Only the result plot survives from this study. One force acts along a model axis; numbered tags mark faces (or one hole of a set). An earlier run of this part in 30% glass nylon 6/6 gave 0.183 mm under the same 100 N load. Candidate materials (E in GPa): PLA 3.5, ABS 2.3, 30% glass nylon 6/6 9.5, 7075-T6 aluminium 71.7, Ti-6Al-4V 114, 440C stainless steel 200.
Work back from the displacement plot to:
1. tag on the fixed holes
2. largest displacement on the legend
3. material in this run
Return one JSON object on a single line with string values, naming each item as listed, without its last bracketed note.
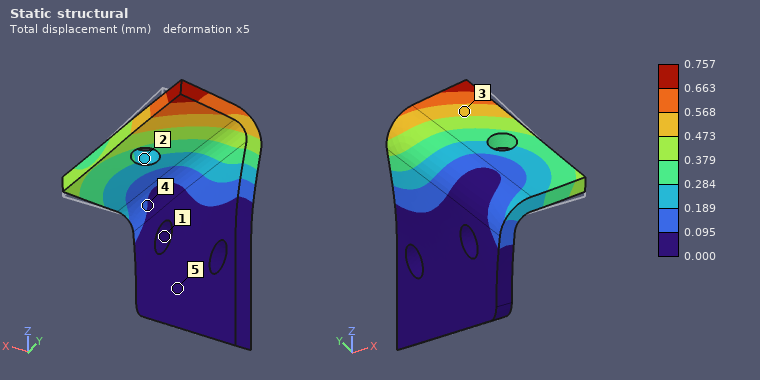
{"tag on the fixed holes": "1", "largest displacement on the legend": "0.757 mm", "material in this run": "ABS"}
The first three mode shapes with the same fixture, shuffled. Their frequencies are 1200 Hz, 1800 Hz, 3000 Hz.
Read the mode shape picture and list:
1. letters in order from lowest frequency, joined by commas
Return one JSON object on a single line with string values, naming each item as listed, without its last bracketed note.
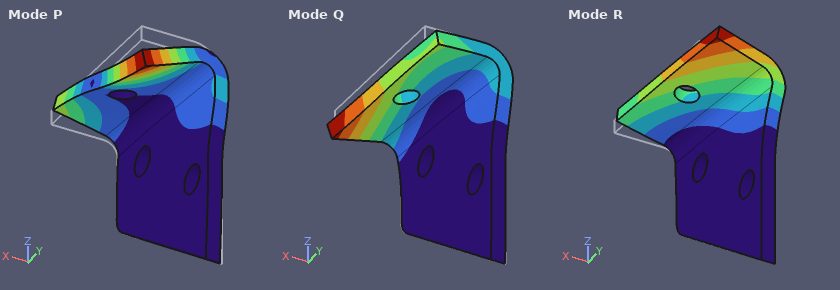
{"letters in order from lowest frequency, joined by commas": "R, Q, P"}
